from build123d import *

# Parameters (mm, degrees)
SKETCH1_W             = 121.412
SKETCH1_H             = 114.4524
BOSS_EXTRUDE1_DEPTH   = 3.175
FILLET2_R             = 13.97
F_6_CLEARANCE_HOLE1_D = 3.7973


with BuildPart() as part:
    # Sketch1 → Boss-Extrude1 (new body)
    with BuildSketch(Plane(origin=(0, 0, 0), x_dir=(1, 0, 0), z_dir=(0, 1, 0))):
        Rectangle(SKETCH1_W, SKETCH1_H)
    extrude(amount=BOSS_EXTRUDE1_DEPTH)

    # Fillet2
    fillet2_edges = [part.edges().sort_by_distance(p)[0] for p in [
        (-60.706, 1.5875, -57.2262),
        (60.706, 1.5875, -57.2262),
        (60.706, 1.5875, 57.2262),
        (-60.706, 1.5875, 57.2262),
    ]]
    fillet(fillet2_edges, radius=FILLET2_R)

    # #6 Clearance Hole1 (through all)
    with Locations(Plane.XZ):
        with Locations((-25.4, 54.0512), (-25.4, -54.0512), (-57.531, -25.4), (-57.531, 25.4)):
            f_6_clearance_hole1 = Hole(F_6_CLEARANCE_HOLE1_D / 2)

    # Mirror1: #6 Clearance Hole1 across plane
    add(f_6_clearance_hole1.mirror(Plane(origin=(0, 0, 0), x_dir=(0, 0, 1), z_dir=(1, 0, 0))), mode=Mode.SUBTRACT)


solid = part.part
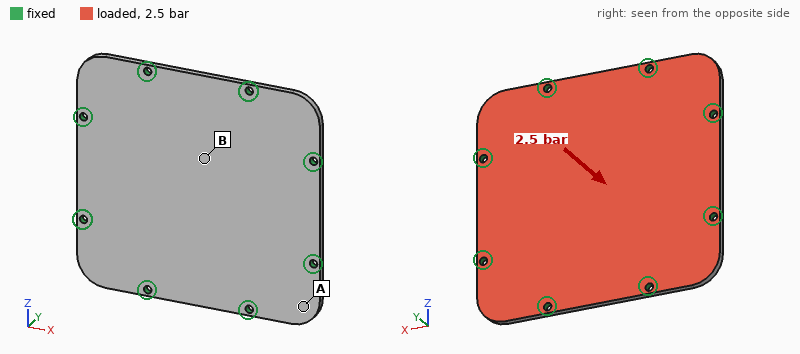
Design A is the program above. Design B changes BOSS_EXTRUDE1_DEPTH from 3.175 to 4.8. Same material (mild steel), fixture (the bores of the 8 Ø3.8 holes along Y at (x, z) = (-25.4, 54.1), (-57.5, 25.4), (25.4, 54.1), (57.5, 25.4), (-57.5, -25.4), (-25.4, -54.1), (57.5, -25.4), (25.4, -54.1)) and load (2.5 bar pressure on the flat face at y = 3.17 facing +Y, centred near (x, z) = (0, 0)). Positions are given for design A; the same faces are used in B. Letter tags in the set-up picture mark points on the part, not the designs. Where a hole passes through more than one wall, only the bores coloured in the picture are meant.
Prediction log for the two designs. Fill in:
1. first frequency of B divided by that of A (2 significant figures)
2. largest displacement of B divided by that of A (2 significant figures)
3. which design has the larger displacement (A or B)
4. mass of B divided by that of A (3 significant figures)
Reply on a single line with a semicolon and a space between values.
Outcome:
1.5; 0.31; A; 1.51
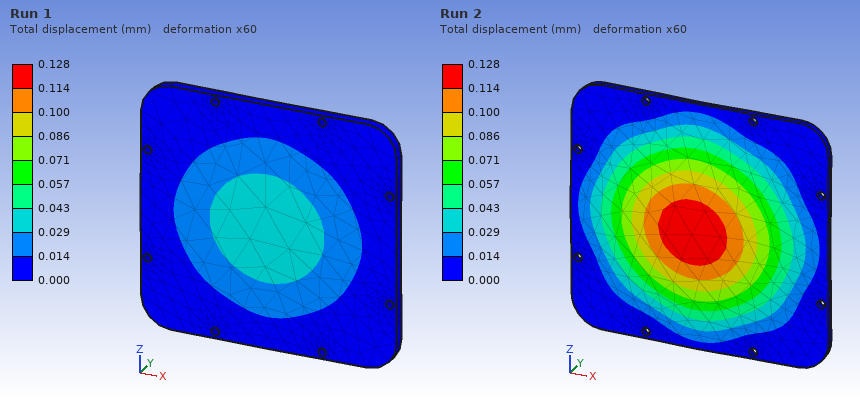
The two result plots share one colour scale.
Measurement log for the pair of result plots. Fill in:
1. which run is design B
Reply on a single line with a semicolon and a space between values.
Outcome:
Run 1
